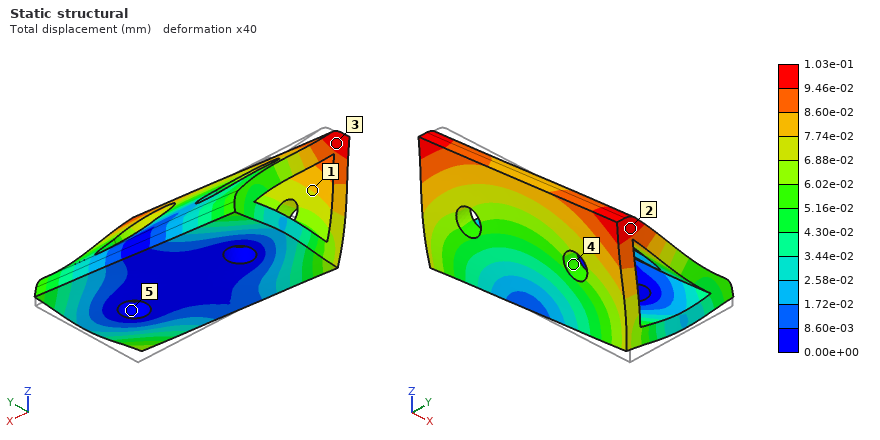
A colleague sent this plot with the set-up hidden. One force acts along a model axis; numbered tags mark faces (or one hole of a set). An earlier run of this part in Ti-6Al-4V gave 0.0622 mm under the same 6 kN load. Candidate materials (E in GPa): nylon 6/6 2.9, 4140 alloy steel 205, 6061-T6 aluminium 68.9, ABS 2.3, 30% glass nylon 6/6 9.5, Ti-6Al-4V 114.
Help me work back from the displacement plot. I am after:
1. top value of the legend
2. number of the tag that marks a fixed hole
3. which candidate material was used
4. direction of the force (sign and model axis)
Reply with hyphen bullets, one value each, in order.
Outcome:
- 1.03e-01 mm
- 5
- 6061-T6 aluminium
- -X
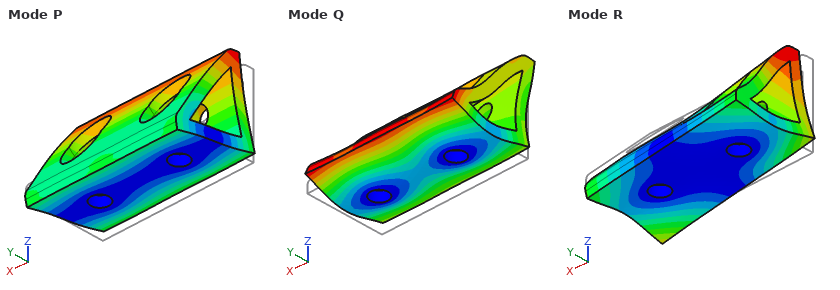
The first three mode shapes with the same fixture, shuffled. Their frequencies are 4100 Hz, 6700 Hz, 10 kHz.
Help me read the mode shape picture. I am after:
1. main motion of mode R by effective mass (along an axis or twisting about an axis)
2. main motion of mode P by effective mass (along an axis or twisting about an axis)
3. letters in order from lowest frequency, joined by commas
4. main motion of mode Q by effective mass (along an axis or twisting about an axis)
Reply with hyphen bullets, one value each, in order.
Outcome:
- along X
- along Y
- P, R, Q
- along Z
